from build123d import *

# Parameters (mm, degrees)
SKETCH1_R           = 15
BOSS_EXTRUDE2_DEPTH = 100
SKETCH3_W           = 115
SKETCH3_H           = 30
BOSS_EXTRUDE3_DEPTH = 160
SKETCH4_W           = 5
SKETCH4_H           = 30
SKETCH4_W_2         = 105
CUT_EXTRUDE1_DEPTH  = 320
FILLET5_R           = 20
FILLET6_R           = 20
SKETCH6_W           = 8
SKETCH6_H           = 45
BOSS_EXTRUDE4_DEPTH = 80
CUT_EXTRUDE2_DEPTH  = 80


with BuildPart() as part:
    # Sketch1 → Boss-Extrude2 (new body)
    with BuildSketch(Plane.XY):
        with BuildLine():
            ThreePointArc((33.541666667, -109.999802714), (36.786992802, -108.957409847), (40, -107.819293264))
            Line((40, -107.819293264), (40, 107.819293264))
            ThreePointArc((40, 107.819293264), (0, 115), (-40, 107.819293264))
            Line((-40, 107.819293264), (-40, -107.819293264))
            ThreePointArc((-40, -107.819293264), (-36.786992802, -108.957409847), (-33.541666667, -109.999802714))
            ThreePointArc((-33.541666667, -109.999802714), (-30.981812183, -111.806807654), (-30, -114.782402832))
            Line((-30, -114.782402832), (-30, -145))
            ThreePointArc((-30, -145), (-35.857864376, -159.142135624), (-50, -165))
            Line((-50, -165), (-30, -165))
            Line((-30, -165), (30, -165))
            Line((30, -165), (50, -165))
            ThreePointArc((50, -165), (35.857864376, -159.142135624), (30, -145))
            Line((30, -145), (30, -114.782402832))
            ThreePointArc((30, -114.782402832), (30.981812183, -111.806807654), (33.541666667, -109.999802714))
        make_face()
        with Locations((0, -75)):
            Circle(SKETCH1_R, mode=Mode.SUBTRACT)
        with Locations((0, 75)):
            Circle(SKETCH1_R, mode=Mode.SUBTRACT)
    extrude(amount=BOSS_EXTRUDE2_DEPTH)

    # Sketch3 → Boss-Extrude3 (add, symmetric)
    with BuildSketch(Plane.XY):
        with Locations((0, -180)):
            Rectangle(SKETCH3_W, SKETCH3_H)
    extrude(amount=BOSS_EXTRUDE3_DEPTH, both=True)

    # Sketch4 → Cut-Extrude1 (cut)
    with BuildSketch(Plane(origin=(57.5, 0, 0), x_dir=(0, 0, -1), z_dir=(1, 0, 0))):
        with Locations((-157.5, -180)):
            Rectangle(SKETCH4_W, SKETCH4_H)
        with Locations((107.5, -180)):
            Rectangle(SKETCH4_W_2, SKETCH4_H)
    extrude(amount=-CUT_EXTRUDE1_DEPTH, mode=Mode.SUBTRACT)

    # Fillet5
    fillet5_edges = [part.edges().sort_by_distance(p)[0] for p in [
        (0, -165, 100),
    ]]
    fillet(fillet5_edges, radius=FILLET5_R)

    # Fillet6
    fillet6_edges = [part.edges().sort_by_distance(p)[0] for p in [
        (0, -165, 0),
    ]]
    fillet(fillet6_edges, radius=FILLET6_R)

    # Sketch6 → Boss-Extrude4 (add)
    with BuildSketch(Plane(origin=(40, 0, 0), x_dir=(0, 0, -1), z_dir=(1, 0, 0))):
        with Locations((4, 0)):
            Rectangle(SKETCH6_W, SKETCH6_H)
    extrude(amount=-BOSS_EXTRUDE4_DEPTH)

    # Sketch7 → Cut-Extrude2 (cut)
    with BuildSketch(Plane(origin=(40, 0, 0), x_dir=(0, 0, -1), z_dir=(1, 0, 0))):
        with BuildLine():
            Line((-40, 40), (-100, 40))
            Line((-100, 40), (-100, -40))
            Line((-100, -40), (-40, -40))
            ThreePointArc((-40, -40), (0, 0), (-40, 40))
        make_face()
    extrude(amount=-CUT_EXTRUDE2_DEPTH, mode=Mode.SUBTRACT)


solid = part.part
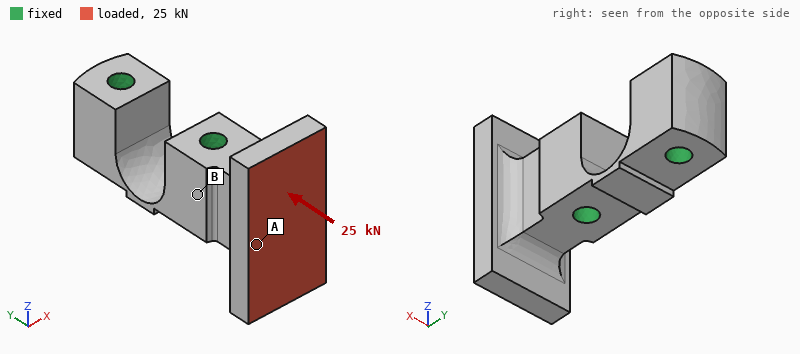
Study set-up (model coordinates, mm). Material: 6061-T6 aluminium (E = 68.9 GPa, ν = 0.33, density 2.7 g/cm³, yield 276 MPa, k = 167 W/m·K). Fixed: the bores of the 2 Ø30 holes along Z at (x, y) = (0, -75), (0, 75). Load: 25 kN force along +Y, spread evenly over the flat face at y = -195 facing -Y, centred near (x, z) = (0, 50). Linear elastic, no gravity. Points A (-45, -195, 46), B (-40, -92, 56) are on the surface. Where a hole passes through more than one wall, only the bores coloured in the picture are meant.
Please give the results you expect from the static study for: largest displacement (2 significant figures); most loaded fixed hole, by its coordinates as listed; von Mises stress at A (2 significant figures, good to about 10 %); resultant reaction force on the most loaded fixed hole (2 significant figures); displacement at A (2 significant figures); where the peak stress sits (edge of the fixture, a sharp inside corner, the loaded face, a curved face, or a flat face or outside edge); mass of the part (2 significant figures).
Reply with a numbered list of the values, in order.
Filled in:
1. 25 µm
2. (0, -75)
3. 5.4 MPa
4. 25 kN
5. 4.1 µm
6. a curved face
7. 5.9 kg
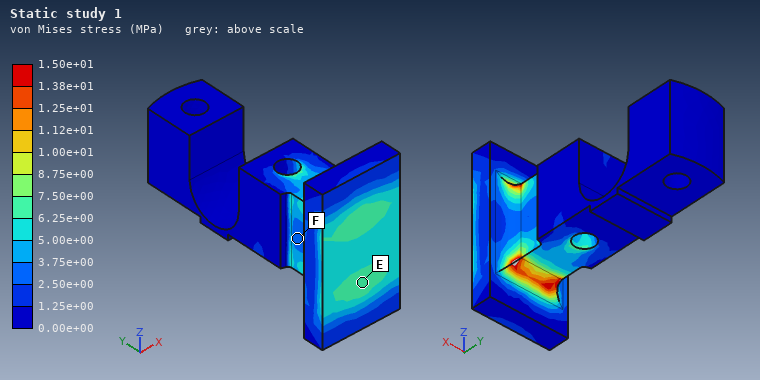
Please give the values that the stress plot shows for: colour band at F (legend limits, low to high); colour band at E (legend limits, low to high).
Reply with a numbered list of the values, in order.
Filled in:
1. 2.50e+00 to 3.75e+00 MPa
2. 6.25e+00 to 7.50e+00 MPa
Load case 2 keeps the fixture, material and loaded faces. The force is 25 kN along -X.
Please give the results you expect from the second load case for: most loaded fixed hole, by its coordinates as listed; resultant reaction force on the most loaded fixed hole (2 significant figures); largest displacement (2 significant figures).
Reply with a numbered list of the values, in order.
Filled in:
1. (0, -75)
2. 27 kN
3. 0.15 mm
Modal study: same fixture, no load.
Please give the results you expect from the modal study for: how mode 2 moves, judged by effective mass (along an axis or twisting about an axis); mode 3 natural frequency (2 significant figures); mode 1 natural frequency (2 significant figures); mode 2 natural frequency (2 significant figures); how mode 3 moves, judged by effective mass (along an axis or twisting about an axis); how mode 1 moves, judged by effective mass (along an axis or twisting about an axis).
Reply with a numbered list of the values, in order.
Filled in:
1. twisting about Y
2. 2300 Hz
3. 1700 Hz
4. 2100 Hz
5. along Z
6. along X
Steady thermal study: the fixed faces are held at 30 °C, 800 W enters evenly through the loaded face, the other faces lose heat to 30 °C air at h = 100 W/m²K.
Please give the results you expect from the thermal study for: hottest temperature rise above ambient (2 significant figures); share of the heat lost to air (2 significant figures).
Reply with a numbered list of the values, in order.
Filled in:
1. 58 K
2. 31 %
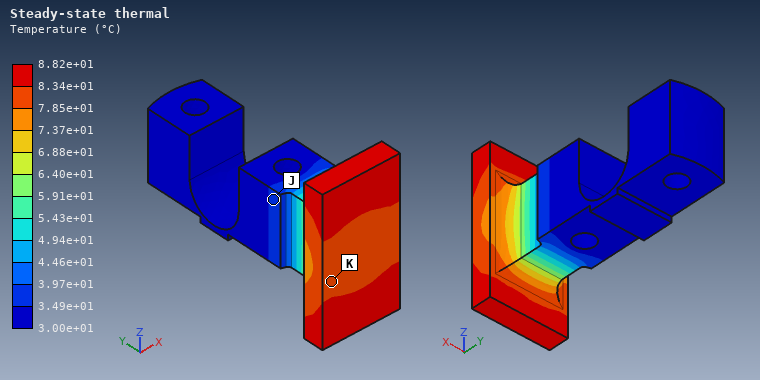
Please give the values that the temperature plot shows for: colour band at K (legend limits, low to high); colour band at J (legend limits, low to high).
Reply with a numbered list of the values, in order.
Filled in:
1. 7.85e+01 to 8.34e+01 °C
2. 3.49e+01 to 3.97e+01 °C
